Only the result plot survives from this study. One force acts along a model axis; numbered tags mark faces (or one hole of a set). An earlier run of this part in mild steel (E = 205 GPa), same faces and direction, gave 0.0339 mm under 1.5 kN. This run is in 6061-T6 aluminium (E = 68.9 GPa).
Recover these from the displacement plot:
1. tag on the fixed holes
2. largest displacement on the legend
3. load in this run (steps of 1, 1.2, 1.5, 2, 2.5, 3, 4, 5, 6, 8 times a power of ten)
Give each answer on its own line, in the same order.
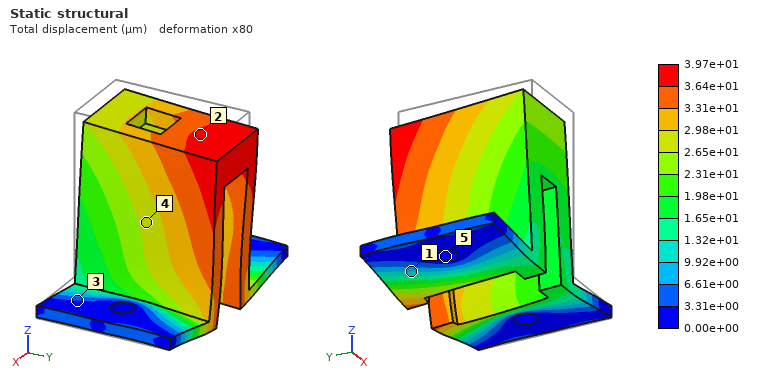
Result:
5
3.97e+01 µm
600 N
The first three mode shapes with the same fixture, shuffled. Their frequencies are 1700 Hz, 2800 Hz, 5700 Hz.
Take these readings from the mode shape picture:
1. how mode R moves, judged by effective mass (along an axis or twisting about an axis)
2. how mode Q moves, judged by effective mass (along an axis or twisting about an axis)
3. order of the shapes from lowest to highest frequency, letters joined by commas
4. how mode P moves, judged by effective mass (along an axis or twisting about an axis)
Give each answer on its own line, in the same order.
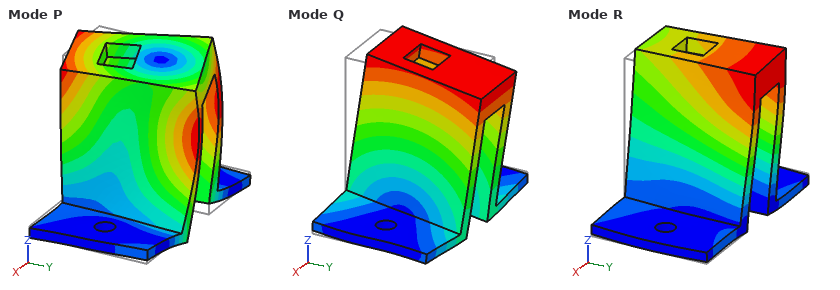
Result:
along X
along Y
Q, R, P
twisting about Z
